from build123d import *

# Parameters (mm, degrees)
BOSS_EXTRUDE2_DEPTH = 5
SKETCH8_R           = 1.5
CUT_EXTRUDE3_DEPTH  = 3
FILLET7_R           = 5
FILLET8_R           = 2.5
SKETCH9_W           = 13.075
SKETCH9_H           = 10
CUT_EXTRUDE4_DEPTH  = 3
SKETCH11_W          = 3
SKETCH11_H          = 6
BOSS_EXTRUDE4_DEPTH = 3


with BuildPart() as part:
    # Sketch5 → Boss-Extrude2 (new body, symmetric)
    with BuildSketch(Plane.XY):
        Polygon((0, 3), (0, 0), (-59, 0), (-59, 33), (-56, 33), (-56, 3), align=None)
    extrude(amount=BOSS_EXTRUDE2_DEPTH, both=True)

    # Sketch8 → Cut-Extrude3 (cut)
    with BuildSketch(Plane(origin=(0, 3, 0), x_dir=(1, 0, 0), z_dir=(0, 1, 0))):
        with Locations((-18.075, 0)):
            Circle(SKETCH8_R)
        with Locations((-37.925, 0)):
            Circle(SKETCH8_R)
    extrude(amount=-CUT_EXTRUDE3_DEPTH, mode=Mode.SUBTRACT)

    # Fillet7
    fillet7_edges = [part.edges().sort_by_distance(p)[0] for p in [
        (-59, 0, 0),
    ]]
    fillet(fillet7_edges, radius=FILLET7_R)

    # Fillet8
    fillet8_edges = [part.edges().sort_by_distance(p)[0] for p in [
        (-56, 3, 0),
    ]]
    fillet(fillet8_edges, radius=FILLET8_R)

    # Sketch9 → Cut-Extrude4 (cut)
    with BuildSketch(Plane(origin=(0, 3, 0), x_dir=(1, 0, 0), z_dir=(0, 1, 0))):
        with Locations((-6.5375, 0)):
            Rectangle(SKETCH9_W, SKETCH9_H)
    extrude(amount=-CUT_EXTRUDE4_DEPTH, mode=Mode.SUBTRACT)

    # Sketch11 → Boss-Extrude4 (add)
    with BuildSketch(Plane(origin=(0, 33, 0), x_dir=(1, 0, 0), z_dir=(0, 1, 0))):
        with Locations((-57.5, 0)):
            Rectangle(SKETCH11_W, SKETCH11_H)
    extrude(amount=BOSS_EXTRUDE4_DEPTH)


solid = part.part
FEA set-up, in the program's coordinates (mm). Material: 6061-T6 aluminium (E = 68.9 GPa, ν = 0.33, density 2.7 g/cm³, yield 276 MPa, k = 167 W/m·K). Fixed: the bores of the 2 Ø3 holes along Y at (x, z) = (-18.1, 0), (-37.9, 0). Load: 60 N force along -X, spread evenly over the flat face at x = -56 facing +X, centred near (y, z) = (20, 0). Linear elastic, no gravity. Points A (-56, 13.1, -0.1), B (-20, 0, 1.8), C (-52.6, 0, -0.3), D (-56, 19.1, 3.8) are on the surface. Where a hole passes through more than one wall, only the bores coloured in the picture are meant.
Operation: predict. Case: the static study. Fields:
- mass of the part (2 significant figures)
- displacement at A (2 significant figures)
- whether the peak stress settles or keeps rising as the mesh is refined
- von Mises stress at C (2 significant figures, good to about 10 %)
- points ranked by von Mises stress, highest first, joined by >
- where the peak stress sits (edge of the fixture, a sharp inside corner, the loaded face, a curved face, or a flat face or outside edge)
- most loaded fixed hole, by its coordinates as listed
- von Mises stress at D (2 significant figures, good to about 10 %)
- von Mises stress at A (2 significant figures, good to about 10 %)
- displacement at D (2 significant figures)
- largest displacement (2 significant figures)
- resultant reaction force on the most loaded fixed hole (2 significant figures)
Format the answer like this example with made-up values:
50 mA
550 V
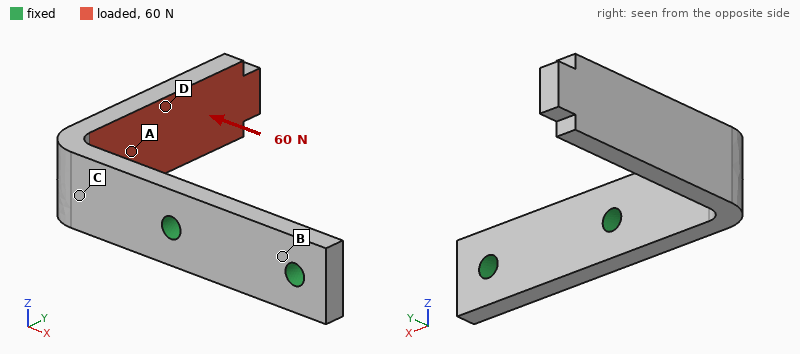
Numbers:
6.1 g
0.20 mm
keeps rising
65 MPa
C > A > D > B
edge of the fixture
(-37.9, 0)
17 MPa
32 MPa
0.30 mm
0.64 mm
56 N
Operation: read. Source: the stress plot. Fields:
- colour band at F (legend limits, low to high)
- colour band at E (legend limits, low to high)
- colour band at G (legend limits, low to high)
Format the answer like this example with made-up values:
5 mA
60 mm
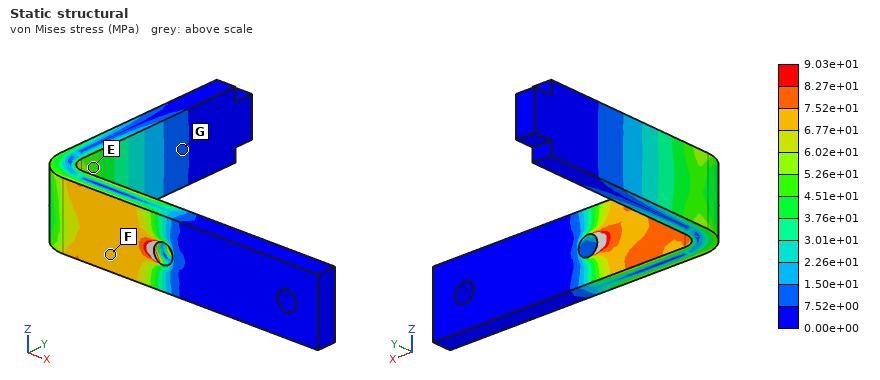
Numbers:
6.77e+01 to 7.52e+01 MPa
4.51e+01 to 5.26e+01 MPa
7.52e+00 to 1.50e+01 MPa
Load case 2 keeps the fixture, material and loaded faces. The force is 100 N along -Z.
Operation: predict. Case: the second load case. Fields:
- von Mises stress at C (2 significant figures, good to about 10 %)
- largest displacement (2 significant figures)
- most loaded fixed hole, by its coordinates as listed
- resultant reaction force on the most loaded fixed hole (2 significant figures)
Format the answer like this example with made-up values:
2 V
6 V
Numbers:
110 MPa
0.62 mm
(-37.9, 0)
150 N
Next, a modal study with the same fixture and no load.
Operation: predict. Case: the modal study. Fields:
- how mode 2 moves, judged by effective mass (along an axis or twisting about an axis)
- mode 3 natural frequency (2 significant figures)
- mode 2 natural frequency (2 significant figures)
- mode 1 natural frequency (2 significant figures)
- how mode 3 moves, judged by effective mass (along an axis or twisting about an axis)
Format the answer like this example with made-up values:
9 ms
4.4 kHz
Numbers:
along Z
3800 Hz
1600 Hz
1200 Hz
along Y
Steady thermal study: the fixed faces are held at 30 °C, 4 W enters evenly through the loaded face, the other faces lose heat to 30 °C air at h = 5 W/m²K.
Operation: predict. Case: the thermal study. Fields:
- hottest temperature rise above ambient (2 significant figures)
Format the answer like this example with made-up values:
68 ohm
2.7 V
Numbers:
28 K
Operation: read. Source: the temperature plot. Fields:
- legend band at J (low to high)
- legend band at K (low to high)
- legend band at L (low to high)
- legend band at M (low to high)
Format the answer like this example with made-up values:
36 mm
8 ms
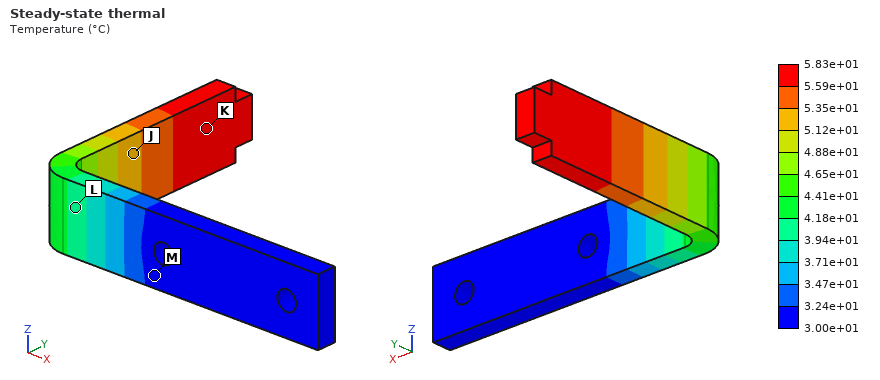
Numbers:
5.12e+01 to 5.35e+01 °C
5.59e+01 to 5.83e+01 °C
3.94e+01 to 4.18e+01 °C
3.00e+01 to 3.24e+01 °C
